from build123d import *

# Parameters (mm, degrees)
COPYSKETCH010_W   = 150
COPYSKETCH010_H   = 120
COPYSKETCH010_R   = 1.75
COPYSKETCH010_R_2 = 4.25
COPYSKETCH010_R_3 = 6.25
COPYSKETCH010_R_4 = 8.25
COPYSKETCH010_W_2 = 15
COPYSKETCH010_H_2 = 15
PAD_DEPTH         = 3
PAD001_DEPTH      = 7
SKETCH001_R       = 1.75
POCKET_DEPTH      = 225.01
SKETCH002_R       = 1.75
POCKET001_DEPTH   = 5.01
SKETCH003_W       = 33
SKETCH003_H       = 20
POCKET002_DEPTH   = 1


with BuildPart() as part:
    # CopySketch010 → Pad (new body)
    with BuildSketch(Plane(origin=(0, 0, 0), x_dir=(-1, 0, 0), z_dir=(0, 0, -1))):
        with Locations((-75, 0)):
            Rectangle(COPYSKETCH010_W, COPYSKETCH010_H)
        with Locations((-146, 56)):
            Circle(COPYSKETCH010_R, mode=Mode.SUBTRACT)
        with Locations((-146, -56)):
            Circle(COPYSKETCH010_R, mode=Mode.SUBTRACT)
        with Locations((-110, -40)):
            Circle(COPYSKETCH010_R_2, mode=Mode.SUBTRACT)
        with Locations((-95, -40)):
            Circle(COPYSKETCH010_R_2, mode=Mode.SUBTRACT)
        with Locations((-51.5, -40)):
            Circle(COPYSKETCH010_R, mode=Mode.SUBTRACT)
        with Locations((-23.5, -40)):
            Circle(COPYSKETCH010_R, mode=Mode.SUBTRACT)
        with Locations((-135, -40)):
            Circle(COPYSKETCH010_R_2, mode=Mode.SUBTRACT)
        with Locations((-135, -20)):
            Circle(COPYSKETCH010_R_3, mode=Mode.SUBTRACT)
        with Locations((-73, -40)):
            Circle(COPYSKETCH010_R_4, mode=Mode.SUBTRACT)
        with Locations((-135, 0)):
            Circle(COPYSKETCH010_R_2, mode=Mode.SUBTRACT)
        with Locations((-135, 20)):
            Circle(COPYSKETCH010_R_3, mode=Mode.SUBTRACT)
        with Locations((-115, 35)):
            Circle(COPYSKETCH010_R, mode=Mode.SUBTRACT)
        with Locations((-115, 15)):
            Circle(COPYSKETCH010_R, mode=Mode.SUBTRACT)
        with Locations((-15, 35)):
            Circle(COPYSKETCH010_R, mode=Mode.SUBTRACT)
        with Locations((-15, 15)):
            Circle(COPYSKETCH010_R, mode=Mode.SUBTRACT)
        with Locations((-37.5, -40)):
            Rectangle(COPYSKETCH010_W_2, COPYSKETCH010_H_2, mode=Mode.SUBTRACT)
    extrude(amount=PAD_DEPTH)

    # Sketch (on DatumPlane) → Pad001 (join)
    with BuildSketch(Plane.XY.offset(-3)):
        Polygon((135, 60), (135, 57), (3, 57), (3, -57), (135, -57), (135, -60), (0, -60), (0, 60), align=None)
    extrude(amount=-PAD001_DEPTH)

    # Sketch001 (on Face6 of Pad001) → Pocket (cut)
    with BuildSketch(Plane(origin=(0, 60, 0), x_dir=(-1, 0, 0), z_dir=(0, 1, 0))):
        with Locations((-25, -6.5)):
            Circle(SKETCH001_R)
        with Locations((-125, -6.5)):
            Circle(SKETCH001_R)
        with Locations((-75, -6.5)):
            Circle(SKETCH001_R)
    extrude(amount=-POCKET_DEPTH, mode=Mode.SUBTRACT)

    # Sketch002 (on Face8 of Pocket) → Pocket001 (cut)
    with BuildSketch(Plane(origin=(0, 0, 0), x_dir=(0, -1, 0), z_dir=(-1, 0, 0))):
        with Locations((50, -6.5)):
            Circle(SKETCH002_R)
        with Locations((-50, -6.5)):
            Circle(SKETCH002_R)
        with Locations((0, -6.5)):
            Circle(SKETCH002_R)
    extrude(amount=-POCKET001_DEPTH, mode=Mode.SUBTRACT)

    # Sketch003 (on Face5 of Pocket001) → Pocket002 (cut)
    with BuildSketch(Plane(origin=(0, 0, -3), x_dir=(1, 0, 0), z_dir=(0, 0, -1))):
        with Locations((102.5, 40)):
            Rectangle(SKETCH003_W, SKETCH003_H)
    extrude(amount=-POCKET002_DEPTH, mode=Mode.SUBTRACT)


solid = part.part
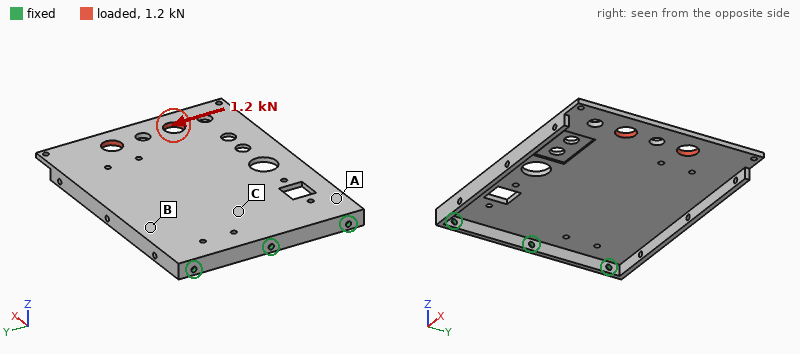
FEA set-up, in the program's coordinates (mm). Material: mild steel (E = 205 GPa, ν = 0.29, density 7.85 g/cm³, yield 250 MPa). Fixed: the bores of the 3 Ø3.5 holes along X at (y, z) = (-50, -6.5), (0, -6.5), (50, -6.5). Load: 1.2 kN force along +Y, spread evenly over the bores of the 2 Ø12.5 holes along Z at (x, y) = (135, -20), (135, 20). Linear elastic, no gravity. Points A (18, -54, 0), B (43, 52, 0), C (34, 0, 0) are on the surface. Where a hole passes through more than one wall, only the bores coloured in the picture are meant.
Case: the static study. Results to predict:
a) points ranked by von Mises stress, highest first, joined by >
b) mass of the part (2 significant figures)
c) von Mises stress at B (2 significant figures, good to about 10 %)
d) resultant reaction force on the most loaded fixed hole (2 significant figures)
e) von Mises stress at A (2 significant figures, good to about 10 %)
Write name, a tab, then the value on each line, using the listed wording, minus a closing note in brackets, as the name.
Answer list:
points ranked by von Mises stress, highest first, joined by >	A > B > C
mass of the part	460 g
von Mises stress at B	12 MPa
resultant reaction force on the most loaded fixed hole	1.6 kN
von Mises stress at A	21 MPa
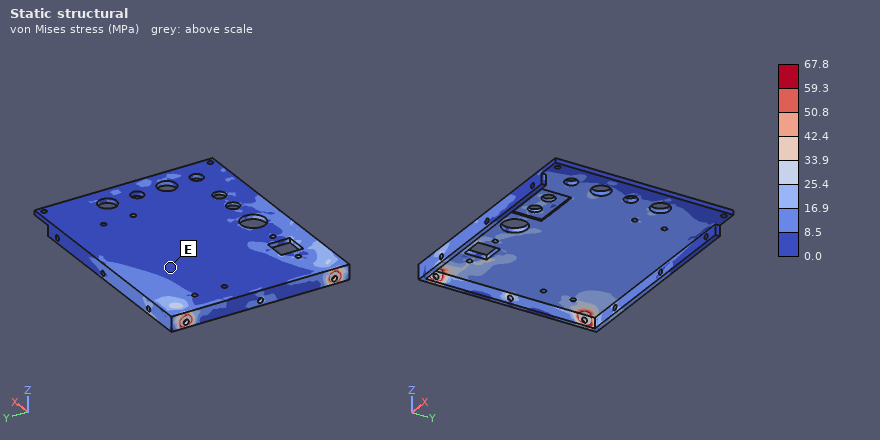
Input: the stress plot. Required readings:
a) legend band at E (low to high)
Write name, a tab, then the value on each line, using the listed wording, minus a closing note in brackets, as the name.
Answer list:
legend band at E	0.0 to 8.5 MPa
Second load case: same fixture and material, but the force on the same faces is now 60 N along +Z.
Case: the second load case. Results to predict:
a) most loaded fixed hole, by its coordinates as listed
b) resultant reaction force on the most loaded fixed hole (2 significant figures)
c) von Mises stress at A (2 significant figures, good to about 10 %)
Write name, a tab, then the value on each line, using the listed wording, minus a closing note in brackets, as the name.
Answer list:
most loaded fixed hole, by its coordinates as listed	(0, -6.5)
resultant reaction force on the most loaded fixed hole	230 N
von Mises stress at A	15 MPa
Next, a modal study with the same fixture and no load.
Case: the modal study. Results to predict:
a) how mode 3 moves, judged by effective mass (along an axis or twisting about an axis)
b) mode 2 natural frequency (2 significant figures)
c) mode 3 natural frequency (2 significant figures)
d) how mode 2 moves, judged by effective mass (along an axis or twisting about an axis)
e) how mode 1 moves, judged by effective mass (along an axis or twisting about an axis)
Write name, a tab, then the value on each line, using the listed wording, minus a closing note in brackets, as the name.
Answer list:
how mode 3 moves, judged by effective mass	along Z
mode 2 natural frequency	350 Hz
mode 3 natural frequency	990 Hz
how mode 2 moves, judged by effective mass	twisting about X
how mode 1 moves, judged by effective mass	along Z
